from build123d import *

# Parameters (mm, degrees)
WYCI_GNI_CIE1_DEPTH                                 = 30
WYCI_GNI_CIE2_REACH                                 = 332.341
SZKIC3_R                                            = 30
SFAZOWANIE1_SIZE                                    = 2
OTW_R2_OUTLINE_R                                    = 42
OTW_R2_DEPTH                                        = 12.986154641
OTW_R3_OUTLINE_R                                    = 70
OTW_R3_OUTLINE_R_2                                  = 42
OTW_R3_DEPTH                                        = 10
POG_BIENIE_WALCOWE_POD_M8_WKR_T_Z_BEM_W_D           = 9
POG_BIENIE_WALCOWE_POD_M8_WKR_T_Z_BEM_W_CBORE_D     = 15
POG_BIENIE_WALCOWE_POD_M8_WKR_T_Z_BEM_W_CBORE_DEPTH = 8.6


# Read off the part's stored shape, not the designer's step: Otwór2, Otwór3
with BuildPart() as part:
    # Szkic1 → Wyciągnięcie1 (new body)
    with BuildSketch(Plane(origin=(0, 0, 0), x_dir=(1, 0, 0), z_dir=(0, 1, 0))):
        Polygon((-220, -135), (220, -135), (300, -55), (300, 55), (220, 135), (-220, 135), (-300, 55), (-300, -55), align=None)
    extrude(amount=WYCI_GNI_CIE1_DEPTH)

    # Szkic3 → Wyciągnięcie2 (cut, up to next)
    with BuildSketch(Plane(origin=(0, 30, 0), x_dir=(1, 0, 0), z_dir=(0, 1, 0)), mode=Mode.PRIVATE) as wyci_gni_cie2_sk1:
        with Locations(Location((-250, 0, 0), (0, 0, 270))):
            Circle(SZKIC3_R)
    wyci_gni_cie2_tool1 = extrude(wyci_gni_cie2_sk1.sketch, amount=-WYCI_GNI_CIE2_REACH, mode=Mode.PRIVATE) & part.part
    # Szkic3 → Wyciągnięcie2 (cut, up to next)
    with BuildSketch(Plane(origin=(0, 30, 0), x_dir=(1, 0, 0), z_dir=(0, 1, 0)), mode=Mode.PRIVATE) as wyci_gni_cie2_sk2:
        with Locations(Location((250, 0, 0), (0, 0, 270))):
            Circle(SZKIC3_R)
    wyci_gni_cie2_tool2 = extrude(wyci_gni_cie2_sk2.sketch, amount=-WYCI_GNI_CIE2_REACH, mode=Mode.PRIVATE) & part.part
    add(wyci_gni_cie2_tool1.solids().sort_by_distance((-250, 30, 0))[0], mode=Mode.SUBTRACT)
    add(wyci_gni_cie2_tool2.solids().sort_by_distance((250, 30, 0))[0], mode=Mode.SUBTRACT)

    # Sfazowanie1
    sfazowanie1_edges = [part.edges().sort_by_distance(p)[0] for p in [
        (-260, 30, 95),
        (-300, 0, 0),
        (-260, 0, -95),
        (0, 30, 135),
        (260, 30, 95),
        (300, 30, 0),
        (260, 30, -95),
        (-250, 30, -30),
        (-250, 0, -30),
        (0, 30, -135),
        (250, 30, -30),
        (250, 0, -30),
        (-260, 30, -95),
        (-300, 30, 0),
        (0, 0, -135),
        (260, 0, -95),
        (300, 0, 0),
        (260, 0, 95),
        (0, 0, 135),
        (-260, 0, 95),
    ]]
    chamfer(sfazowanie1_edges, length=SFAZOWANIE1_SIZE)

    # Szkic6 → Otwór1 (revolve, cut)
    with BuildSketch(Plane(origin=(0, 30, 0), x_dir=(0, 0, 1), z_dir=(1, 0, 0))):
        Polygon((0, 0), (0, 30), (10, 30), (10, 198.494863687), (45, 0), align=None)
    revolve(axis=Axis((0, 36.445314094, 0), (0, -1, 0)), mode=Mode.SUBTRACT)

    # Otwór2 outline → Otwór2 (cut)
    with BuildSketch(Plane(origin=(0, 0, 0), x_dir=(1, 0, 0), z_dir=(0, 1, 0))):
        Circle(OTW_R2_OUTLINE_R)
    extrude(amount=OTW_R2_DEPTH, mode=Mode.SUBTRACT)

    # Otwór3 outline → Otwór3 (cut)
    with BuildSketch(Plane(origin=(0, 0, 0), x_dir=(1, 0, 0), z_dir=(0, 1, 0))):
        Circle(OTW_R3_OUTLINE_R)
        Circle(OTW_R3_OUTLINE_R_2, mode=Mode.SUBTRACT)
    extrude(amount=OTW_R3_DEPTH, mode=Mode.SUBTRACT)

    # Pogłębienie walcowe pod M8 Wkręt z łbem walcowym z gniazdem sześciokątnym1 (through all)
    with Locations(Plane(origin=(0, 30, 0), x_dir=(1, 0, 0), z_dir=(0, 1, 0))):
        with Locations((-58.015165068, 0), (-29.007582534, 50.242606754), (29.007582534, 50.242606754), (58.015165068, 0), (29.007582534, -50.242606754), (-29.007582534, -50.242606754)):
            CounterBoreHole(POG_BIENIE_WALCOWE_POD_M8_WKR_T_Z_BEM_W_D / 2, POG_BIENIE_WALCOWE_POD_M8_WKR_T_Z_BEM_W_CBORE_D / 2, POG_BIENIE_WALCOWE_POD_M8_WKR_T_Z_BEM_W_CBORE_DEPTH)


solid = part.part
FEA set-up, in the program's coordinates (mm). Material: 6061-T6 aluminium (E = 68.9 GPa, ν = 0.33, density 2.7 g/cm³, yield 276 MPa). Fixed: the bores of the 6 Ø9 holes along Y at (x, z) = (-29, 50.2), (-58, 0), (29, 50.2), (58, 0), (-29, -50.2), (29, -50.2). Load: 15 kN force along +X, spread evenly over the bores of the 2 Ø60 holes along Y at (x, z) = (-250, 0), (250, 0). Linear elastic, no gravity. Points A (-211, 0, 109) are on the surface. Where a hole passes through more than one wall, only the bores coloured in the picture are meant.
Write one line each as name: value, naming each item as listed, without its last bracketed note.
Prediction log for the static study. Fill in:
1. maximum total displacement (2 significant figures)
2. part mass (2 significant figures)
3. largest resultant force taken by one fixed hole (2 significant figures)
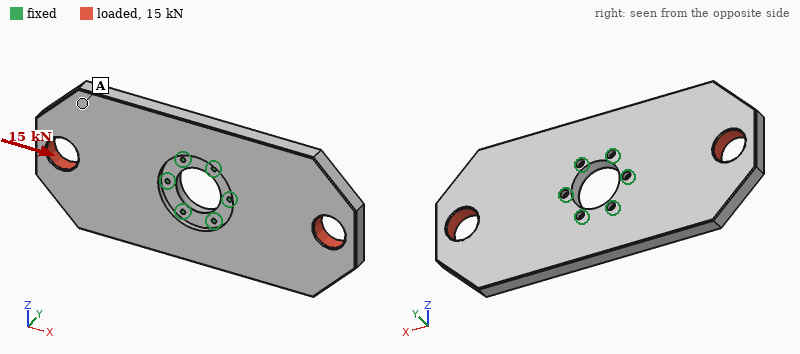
maximum total displacement: 14 µm
part mass: 11 kg
largest resultant force taken by one fixed hole: 2.5 kN
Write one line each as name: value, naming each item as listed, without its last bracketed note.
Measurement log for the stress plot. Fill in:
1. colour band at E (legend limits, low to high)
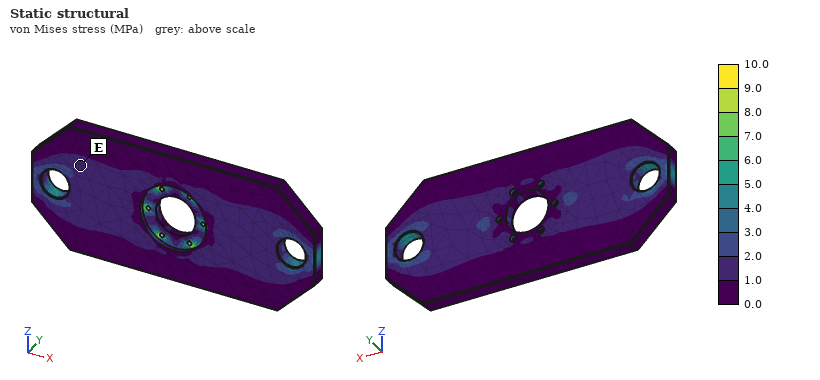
colour band at E: 1.0 to 2.0 MPa
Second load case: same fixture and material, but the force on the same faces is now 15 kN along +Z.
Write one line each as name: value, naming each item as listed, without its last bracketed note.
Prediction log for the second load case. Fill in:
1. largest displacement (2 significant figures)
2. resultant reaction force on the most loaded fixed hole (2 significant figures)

largest displacement: 28 µm
resultant reaction force on the most loaded fixed hole: 3.9 kN
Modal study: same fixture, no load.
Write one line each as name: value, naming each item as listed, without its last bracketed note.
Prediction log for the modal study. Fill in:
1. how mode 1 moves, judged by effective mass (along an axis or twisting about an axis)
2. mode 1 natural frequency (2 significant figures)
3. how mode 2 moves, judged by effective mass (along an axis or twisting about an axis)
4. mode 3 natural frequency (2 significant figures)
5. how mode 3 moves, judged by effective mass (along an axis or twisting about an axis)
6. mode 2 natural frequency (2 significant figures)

how mode 1 moves, judged by effective mass: twisting about Z
mode 1 natural frequency: 300 Hz
how mode 2 moves, judged by effective mass: along Y
mode 3 natural frequency: 650 Hz
how mode 3 moves, judged by effective mass: twisting about X
mode 2 natural frequency: 330 Hz
